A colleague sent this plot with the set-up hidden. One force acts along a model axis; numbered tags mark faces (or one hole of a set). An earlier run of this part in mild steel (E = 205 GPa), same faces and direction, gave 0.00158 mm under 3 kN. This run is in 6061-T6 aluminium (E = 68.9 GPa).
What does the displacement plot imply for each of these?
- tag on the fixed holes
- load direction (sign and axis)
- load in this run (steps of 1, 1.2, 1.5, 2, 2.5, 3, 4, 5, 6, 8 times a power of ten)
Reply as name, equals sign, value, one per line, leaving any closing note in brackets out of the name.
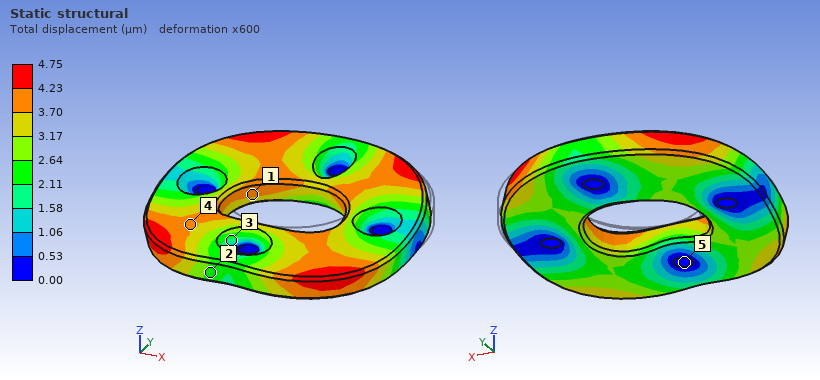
tag on the fixed holes = 5
load direction = -Y
load in this run = 3 kN
